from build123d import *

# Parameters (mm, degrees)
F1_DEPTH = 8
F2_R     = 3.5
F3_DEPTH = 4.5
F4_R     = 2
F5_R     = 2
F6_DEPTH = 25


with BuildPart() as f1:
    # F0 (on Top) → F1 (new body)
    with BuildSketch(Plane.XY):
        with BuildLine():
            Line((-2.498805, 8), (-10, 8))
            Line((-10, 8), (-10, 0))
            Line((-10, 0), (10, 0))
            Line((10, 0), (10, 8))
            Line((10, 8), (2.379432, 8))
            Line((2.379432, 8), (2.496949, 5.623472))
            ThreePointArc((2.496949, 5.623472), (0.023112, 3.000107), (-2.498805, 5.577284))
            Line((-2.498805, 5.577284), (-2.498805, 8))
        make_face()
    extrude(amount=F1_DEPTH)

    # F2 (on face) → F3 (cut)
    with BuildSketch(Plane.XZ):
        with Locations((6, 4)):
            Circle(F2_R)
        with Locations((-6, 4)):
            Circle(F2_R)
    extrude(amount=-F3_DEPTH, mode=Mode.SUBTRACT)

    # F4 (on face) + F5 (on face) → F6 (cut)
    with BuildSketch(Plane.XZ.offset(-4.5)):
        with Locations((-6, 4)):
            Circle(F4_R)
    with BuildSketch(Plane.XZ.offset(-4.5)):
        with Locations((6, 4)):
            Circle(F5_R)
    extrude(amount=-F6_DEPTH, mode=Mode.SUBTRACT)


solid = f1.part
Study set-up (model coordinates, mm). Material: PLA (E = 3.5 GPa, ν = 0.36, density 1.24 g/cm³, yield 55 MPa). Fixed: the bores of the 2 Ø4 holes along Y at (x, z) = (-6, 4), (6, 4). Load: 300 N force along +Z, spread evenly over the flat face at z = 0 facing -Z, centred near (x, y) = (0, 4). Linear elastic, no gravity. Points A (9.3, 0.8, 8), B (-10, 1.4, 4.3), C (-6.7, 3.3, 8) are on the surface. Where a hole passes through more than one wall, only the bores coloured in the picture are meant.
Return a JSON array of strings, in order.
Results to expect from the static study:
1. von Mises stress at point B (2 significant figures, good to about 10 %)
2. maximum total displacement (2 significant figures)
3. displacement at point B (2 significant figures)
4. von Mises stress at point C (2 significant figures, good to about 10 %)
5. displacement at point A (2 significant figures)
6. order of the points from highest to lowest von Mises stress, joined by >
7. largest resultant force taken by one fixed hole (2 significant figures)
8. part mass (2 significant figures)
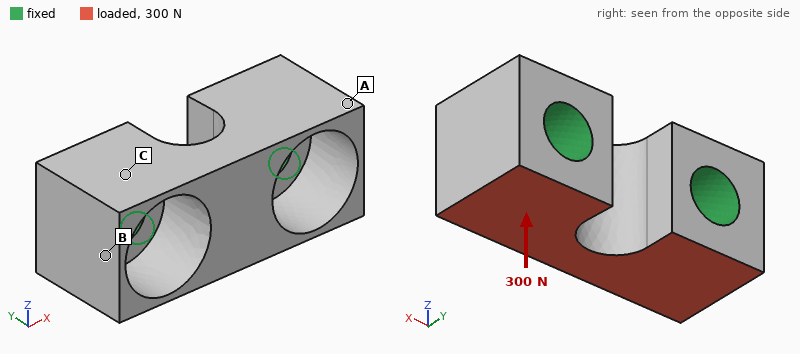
["9.3 MPa", "94 µm", "37 µm", "5.5 MPa", "22 µm", "B > C > A", "150 N", "0.83 g"]
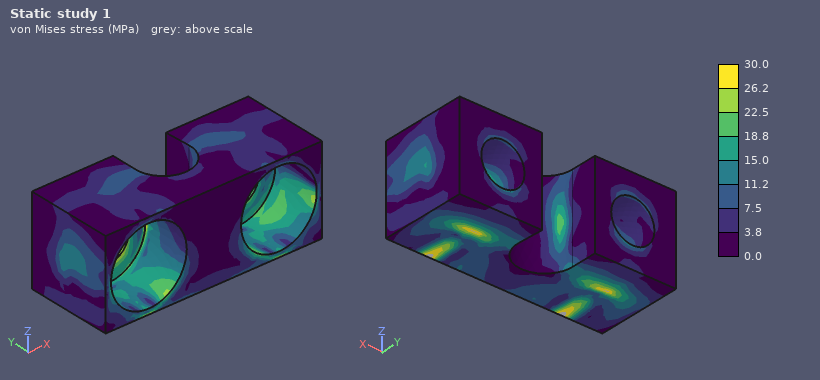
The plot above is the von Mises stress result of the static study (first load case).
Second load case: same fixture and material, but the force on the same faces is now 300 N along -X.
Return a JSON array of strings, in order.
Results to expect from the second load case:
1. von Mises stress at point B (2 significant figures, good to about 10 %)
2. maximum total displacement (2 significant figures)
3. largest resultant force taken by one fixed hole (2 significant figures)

["4.1 MPa", "61 µm", "160 N"]
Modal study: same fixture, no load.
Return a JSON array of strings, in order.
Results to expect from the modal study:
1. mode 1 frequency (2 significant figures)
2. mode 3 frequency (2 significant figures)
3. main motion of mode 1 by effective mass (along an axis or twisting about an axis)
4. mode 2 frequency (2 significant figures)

["17 kHz", "24 kHz", "along Z", "23 kHz"]
